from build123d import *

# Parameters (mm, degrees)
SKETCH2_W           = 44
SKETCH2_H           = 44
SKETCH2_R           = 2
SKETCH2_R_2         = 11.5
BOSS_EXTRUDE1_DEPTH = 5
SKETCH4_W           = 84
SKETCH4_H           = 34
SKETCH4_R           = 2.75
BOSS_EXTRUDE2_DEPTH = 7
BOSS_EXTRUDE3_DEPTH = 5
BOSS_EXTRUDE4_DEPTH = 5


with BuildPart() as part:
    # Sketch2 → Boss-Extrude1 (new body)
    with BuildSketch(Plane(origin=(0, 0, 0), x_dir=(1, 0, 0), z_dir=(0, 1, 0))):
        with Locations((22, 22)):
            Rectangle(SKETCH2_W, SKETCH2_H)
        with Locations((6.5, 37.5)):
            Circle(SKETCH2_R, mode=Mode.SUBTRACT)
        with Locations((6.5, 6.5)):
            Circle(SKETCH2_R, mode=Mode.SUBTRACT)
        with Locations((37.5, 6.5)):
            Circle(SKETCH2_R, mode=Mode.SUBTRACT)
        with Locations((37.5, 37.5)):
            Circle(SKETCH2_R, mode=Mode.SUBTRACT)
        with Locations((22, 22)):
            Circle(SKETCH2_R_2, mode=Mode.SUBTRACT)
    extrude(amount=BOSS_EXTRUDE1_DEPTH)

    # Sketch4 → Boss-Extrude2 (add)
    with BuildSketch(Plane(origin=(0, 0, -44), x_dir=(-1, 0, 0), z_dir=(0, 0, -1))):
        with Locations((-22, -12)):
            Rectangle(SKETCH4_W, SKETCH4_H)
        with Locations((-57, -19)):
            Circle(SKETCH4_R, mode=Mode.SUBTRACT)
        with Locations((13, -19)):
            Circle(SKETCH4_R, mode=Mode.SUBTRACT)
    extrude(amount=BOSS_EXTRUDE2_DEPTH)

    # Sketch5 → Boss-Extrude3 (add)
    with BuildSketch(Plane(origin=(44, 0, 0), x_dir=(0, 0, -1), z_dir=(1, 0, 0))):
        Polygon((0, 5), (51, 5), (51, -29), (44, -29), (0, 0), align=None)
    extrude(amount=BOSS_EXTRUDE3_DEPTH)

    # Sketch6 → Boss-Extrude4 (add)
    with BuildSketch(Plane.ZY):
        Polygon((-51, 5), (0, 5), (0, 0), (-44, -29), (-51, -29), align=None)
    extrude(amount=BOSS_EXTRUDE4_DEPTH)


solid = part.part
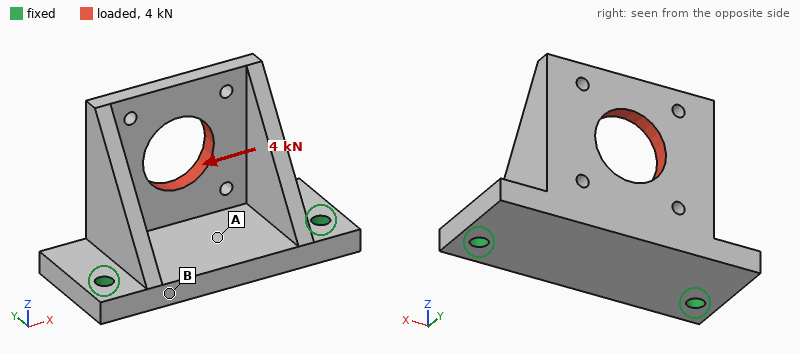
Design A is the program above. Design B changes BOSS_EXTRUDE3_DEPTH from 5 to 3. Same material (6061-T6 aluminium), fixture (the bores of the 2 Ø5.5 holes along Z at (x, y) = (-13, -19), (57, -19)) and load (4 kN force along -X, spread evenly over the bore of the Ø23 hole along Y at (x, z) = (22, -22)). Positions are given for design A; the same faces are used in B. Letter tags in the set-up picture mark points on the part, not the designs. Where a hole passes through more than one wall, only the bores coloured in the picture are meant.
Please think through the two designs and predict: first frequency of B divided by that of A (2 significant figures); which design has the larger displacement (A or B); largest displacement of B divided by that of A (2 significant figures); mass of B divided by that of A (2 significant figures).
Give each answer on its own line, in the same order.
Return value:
0.99
B
1.2
0.95
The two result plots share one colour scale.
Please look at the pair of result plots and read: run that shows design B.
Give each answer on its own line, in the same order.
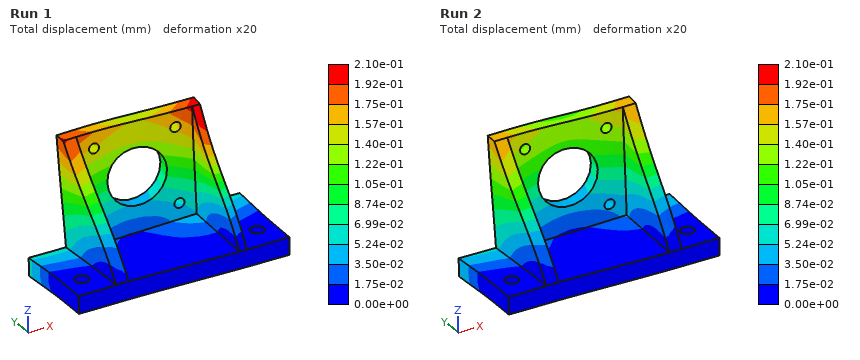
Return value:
Run 1
